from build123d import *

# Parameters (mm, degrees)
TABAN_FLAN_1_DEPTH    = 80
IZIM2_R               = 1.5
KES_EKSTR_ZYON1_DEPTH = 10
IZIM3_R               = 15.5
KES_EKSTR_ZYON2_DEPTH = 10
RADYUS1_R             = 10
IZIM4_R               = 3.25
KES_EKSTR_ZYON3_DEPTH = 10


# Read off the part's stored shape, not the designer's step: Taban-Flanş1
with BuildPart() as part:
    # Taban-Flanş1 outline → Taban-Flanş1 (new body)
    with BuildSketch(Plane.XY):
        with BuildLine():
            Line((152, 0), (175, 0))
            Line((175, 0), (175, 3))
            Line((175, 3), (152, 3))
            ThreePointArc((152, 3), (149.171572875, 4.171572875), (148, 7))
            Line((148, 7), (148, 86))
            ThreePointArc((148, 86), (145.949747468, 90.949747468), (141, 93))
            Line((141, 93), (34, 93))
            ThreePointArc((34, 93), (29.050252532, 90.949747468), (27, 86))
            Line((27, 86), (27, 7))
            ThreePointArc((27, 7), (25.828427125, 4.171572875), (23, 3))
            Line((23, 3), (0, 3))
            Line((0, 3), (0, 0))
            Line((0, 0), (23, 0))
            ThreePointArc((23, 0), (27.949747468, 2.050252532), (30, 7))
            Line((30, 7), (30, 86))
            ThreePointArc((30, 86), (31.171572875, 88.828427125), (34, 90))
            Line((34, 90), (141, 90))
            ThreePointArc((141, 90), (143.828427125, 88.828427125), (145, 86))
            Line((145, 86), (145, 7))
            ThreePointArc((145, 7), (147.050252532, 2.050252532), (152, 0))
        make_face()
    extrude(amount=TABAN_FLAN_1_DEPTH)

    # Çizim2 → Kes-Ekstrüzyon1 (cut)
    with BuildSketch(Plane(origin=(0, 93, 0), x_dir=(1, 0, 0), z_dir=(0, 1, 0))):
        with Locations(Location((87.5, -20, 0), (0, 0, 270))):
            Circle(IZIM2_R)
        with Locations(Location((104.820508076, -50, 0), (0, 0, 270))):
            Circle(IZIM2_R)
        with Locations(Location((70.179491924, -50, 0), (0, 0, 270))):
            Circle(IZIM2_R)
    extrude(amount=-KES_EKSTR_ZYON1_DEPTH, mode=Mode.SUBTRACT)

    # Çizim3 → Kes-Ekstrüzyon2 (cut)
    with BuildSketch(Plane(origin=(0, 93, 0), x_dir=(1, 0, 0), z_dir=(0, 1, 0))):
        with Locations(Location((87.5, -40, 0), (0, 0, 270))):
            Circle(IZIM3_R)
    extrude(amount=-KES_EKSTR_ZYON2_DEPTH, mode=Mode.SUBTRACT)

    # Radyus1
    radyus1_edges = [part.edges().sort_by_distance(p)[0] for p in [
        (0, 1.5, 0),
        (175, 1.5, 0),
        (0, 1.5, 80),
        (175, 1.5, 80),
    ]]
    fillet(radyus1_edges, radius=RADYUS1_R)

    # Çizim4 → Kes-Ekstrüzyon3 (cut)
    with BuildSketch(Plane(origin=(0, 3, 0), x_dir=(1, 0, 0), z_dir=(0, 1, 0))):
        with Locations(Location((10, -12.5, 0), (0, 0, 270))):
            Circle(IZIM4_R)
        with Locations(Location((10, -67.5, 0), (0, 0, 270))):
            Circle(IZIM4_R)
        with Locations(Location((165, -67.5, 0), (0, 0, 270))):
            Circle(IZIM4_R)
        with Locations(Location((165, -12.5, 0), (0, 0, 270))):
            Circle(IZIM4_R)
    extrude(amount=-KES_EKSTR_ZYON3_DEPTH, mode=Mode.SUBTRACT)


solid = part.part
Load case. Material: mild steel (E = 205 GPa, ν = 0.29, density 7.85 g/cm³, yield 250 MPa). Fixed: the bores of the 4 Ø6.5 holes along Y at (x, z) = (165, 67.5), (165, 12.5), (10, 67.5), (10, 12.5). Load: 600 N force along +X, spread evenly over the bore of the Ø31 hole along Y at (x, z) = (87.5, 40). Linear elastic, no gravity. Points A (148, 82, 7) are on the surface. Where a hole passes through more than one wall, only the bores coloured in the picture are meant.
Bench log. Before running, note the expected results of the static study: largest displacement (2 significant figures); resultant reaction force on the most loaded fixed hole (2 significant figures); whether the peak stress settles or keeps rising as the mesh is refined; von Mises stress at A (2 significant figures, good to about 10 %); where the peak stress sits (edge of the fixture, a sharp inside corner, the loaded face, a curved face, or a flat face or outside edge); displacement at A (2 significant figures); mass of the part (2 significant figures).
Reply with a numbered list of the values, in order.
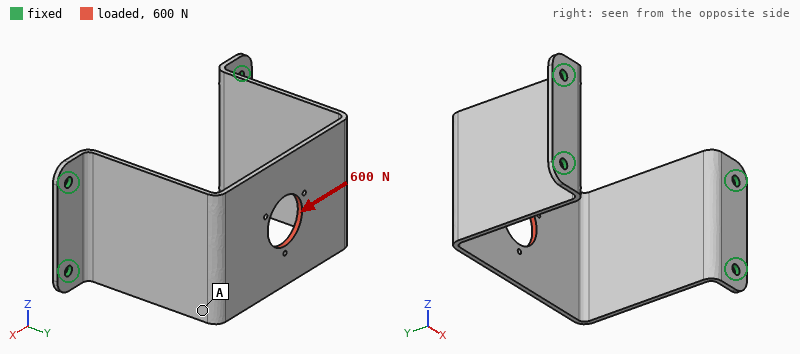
1. 0.92 mm
2. 200 N
3. keeps rising
4. 76 MPa
5. edge of the fixture
6. 0.85 mm
7. 630 g
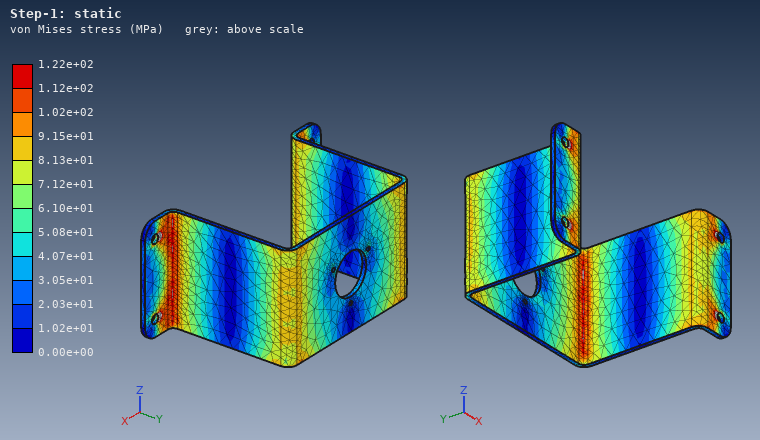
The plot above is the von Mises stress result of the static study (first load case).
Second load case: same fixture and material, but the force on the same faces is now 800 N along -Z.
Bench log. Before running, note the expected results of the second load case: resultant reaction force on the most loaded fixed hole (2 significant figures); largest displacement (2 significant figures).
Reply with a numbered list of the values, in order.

1. 670 N
2. 0.16 mm
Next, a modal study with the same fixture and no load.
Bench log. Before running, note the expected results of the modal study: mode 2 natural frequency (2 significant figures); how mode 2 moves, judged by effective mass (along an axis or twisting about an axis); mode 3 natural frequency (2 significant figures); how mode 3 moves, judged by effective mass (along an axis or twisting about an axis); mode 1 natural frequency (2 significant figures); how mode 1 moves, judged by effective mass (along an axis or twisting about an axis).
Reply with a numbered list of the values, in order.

1. 630 Hz
2. along Z
3. 700 Hz
4. twisting about Y
5. 230 Hz
6. along X
